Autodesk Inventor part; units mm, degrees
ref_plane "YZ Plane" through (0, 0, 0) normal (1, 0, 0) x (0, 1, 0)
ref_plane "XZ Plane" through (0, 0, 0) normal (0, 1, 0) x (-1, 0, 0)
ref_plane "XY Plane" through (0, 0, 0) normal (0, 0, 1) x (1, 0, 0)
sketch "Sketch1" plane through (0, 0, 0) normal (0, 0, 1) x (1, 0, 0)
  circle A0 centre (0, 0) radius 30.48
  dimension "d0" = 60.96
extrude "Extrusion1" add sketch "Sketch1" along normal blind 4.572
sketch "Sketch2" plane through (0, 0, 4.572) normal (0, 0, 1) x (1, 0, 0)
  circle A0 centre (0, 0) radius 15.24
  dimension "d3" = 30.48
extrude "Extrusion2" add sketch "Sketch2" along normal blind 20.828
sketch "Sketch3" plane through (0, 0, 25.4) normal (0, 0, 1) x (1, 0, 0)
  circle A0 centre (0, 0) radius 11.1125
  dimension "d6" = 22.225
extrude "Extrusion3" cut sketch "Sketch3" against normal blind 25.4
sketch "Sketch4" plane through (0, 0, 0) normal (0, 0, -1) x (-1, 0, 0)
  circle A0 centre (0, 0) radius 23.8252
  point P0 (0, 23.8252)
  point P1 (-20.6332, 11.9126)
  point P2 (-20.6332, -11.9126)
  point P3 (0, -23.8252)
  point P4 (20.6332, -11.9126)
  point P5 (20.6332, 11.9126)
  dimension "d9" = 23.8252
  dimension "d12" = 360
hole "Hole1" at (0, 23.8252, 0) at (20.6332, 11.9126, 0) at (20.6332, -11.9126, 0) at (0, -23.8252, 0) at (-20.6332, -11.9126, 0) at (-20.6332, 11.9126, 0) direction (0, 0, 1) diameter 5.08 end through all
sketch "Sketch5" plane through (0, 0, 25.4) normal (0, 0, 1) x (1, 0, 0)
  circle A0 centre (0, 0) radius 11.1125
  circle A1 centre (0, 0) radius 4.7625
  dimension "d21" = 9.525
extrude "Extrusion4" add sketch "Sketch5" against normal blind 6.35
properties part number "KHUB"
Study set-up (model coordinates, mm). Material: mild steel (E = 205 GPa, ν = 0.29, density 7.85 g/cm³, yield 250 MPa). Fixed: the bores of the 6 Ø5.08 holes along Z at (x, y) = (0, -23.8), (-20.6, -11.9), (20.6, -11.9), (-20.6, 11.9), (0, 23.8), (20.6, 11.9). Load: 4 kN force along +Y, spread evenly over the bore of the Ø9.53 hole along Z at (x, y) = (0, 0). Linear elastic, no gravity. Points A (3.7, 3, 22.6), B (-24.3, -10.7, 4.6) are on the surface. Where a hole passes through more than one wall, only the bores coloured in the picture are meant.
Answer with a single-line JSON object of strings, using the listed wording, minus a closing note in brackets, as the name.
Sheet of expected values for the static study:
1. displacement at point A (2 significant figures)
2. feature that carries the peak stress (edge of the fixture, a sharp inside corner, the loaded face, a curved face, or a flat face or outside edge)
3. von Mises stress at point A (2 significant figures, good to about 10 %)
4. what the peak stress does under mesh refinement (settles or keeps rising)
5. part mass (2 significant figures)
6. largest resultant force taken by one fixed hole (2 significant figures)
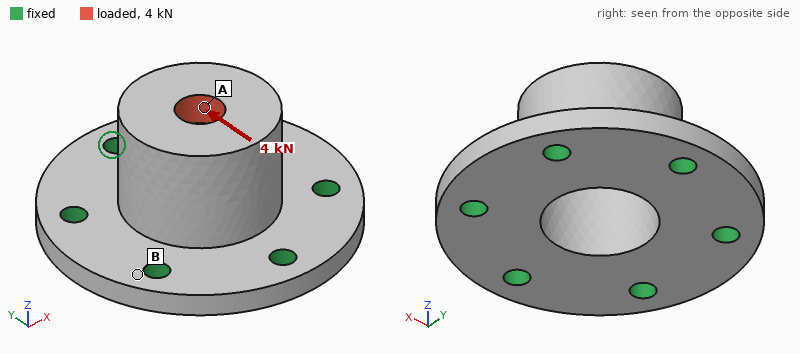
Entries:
{"displacement at point A": "15 µm", "feature that carries the peak stress": "edge of the fixture", "von Mises stress at point A": "35 MPa", "what the peak stress does under mesh refinement": "keeps rising", "part mass": "160 g", "largest resultant force taken by one fixed hole": "1.7 kN"}
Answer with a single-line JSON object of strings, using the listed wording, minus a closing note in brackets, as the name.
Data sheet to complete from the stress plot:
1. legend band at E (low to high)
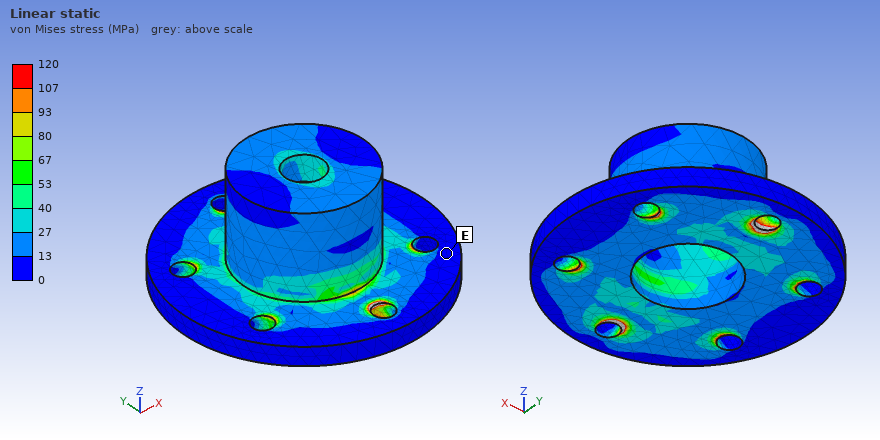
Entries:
{"legend band at E": "0 to 13 MPa"}
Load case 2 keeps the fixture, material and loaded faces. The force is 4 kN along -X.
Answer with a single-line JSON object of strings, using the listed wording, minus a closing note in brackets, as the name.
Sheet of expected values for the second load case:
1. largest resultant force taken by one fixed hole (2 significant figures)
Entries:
{"largest resultant force taken by one fixed hole": "1.5 kN"}
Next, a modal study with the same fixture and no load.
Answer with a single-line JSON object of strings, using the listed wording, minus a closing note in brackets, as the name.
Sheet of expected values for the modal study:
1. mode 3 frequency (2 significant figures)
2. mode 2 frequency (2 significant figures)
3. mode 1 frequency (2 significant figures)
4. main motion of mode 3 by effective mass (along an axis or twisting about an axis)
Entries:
{"mode 3 frequency": "16 kHz", "mode 2 frequency": "12 kHz", "mode 1 frequency": "12 kHz", "main motion of mode 3 by effective mass": "along Z"}
